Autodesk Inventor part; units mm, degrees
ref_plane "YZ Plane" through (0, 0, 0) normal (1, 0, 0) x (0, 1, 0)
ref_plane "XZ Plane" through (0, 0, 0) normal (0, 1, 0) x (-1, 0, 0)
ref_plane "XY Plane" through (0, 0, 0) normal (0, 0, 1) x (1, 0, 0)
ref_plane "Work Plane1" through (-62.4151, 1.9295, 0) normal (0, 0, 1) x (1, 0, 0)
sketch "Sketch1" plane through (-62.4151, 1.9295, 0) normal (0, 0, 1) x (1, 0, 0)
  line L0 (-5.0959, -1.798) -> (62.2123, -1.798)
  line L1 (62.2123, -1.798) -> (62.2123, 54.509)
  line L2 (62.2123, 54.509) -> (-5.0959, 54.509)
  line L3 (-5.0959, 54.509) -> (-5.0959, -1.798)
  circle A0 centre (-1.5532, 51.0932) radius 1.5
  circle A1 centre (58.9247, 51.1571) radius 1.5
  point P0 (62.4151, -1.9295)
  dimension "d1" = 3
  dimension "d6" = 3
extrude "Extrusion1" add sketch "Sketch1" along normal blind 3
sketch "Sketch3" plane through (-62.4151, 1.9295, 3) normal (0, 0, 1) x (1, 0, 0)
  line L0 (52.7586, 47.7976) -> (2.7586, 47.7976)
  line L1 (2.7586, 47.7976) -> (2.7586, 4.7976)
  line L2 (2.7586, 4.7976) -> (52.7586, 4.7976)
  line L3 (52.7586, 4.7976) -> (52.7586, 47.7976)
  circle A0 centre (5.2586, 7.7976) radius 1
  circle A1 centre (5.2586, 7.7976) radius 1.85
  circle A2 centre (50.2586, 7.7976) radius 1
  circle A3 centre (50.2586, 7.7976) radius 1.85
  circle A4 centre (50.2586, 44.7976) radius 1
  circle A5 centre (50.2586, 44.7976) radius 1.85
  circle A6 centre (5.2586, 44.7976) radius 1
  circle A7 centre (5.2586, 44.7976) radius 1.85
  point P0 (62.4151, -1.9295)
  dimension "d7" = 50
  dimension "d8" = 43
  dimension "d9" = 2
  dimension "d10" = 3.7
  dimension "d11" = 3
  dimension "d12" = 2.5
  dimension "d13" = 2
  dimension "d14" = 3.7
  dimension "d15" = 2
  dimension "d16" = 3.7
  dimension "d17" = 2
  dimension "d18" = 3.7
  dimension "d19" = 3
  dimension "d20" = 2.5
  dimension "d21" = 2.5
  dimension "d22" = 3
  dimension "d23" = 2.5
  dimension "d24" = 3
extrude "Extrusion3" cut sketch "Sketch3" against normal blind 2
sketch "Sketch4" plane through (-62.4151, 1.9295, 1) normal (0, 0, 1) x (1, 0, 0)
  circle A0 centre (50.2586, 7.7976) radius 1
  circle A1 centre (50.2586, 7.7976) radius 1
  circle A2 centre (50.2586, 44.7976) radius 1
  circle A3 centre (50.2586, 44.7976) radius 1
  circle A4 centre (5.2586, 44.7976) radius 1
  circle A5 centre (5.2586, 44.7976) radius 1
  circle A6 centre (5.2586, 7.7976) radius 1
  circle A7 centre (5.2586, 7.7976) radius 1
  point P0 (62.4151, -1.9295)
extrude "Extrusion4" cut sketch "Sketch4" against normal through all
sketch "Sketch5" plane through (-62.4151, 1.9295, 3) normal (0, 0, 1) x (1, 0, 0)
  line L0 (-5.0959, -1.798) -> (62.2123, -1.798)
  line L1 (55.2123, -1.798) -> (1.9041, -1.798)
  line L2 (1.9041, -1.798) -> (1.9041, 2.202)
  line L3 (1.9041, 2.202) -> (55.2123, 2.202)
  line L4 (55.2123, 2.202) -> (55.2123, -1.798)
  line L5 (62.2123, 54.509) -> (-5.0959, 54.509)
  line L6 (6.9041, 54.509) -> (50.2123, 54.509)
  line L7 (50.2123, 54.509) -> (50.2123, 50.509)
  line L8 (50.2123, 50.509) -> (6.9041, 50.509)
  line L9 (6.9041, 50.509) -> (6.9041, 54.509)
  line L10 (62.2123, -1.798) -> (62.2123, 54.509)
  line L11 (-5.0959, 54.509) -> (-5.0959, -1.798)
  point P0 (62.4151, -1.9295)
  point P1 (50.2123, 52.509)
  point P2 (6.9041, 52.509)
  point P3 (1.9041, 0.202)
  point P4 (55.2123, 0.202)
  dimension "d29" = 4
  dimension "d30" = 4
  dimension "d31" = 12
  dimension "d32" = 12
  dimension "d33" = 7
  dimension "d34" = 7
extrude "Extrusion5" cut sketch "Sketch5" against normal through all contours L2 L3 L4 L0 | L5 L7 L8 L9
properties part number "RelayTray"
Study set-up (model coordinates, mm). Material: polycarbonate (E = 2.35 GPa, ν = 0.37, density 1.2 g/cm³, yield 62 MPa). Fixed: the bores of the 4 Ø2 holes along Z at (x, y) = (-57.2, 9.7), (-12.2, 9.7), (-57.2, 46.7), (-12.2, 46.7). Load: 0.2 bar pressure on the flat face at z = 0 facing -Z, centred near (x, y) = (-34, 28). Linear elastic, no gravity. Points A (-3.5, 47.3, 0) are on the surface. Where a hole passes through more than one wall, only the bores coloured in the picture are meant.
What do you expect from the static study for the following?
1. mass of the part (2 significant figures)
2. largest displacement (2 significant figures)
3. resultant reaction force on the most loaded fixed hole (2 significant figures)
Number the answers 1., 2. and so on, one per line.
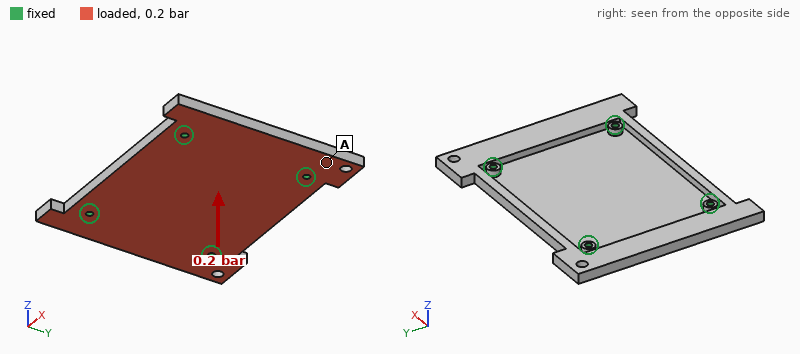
1. 7.1 g
2. 0.93 mm
3. 18 N
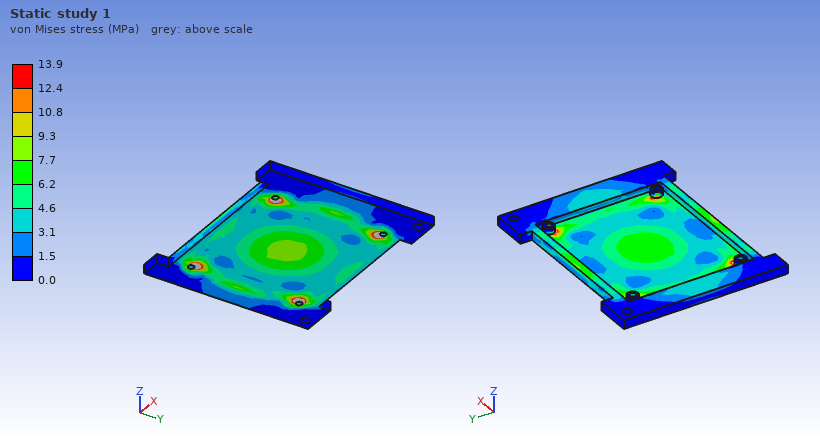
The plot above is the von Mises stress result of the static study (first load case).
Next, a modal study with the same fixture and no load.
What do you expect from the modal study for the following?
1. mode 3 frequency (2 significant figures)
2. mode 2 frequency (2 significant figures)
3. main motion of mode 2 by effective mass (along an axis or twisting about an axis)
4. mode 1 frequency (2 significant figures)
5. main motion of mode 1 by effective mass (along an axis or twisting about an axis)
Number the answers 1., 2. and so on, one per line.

1. 1400 Hz
2. 1200 Hz
3. along Z
4. 810 Hz
5. along Z
